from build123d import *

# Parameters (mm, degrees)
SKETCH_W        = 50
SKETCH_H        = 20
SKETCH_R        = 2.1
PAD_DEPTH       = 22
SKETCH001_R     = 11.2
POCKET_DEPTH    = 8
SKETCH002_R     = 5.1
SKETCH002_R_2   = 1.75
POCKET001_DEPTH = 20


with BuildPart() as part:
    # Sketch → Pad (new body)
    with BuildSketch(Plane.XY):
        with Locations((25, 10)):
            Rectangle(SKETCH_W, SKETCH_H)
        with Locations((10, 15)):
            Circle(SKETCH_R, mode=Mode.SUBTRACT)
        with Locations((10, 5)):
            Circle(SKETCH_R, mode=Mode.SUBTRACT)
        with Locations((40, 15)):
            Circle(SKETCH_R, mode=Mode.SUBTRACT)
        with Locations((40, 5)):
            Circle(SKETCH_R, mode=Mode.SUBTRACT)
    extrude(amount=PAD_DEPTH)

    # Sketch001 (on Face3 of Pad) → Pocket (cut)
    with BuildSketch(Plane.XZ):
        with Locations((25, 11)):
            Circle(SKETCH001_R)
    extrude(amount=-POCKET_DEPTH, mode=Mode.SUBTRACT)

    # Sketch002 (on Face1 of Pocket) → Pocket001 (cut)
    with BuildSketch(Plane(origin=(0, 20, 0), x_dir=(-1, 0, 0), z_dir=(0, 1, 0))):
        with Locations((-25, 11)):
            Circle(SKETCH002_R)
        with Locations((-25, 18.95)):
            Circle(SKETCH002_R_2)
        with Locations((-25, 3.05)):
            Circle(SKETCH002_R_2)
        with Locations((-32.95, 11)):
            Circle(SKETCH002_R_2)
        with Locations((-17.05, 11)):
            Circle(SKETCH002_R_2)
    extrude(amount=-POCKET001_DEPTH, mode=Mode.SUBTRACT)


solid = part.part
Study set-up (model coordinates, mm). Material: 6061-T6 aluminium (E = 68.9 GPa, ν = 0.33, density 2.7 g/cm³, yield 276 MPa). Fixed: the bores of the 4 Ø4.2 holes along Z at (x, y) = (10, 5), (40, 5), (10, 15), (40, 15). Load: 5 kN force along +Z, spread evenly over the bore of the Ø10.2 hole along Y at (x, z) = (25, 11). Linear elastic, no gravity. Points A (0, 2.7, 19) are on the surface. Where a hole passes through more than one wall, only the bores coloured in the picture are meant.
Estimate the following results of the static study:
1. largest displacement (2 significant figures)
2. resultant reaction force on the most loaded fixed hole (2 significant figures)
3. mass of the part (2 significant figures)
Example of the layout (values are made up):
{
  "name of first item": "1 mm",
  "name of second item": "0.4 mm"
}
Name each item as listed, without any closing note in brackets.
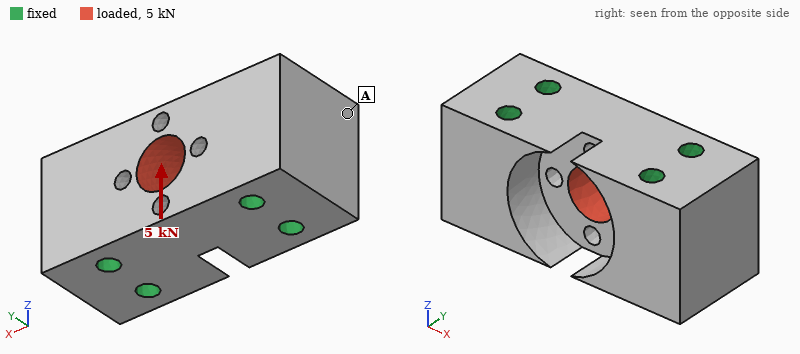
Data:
{
  "largest displacement": "8.9 µm",
  "resultant reaction force on the most loaded fixed hole": "1.9 kN",
  "mass of the part": "44 g"
}
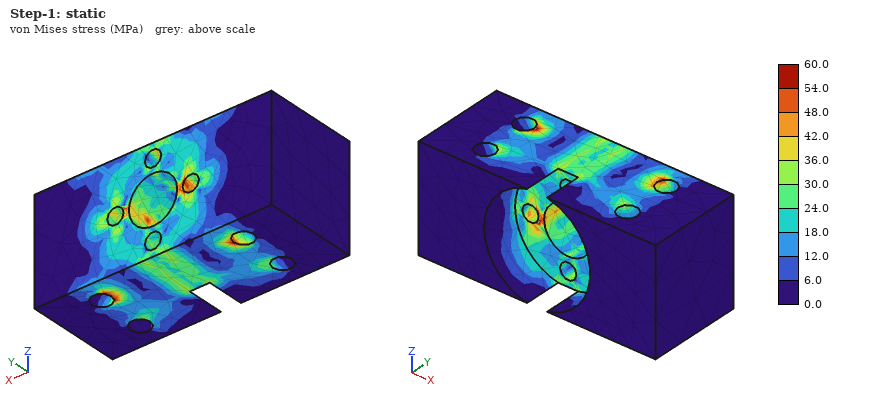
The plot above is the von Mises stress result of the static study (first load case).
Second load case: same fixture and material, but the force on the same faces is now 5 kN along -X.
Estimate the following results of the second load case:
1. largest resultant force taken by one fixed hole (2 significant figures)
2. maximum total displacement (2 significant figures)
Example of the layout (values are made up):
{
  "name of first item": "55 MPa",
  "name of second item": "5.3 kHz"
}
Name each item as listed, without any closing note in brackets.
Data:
{
  "largest resultant force taken by one fixed hole": "2.0 kN",
  "maximum total displacement": "3.4 µm"
}
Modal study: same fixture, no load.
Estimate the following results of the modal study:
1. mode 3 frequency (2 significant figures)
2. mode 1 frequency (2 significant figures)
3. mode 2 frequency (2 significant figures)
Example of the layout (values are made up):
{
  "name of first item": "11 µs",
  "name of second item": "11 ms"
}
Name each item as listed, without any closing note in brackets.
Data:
{
  "mode 3 frequency": "58 kHz",
  "mode 1 frequency": "54 kHz",
  "mode 2 frequency": "54 kHz"
}
